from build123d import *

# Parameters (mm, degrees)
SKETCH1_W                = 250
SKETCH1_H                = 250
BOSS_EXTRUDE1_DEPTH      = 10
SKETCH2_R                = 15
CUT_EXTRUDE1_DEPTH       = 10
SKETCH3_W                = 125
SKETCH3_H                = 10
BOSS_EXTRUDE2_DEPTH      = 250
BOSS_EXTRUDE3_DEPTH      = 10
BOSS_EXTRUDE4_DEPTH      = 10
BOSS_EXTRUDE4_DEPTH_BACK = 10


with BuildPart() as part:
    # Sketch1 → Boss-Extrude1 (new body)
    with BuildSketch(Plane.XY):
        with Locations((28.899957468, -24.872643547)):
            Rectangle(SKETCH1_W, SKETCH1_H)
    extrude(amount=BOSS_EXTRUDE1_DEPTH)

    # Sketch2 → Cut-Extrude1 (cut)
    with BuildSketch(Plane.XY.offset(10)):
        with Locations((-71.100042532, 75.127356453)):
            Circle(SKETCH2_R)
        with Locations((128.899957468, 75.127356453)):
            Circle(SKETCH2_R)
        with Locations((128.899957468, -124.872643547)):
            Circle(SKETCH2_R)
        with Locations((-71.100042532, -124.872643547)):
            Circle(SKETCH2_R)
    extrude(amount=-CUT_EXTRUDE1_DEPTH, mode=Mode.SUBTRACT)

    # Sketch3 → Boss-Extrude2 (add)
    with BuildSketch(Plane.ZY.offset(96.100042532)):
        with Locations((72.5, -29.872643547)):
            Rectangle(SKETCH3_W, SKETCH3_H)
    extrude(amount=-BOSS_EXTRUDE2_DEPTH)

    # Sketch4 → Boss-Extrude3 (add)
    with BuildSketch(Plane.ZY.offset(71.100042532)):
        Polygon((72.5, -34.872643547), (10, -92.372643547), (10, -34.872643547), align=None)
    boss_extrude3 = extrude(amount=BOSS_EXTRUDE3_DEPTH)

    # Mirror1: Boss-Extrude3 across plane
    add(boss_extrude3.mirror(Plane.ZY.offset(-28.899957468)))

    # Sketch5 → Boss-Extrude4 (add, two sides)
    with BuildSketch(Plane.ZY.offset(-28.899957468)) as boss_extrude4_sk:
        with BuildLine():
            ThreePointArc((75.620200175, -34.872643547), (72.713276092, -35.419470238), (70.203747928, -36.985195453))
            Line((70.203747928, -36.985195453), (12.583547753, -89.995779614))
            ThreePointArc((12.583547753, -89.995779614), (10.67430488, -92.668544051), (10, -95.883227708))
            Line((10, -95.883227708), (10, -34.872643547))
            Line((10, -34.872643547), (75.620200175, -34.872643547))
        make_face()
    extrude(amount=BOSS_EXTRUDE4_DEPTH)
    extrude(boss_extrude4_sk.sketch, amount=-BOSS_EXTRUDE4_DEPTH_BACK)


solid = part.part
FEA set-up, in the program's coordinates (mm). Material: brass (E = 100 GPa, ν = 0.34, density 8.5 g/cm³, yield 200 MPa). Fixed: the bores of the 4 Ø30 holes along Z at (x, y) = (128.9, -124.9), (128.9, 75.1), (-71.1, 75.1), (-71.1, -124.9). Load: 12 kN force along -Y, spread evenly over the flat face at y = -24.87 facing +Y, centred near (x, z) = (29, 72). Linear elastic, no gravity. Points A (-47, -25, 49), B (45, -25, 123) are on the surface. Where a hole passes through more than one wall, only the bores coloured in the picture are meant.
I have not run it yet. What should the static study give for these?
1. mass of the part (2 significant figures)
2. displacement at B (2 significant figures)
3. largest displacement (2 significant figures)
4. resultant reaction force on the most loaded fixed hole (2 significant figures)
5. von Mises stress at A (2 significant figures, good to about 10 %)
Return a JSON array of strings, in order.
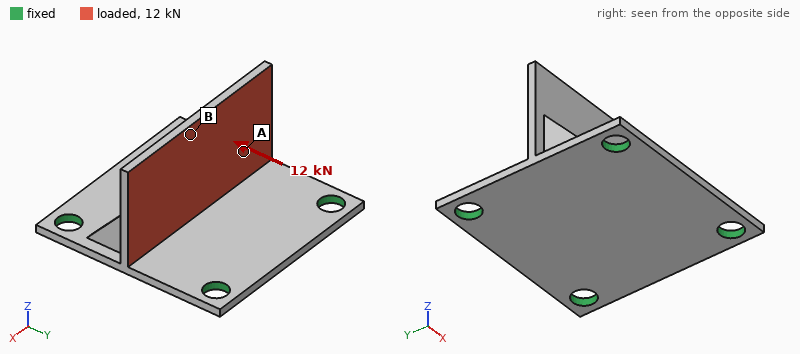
["8.3 kg", "0.60 mm", "0.68 mm", "4.7 kN", "29 MPa"]
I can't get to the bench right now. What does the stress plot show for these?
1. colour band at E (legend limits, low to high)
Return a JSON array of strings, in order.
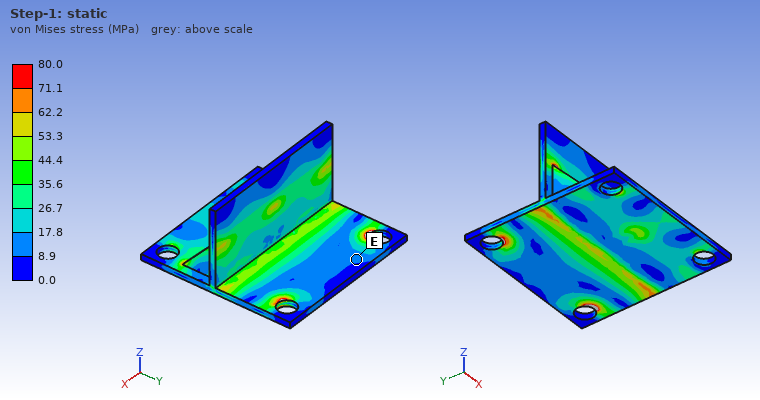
["8.9 to 17.8 MPa"]
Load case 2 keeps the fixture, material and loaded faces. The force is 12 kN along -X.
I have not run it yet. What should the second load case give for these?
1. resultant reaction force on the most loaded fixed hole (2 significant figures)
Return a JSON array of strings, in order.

["5.0 kN"]
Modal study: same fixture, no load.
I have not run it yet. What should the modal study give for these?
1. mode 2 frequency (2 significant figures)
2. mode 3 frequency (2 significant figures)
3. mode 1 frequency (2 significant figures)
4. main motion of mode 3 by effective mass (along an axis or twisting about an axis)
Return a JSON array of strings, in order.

["560 Hz", "740 Hz", "450 Hz", "along Z"]
